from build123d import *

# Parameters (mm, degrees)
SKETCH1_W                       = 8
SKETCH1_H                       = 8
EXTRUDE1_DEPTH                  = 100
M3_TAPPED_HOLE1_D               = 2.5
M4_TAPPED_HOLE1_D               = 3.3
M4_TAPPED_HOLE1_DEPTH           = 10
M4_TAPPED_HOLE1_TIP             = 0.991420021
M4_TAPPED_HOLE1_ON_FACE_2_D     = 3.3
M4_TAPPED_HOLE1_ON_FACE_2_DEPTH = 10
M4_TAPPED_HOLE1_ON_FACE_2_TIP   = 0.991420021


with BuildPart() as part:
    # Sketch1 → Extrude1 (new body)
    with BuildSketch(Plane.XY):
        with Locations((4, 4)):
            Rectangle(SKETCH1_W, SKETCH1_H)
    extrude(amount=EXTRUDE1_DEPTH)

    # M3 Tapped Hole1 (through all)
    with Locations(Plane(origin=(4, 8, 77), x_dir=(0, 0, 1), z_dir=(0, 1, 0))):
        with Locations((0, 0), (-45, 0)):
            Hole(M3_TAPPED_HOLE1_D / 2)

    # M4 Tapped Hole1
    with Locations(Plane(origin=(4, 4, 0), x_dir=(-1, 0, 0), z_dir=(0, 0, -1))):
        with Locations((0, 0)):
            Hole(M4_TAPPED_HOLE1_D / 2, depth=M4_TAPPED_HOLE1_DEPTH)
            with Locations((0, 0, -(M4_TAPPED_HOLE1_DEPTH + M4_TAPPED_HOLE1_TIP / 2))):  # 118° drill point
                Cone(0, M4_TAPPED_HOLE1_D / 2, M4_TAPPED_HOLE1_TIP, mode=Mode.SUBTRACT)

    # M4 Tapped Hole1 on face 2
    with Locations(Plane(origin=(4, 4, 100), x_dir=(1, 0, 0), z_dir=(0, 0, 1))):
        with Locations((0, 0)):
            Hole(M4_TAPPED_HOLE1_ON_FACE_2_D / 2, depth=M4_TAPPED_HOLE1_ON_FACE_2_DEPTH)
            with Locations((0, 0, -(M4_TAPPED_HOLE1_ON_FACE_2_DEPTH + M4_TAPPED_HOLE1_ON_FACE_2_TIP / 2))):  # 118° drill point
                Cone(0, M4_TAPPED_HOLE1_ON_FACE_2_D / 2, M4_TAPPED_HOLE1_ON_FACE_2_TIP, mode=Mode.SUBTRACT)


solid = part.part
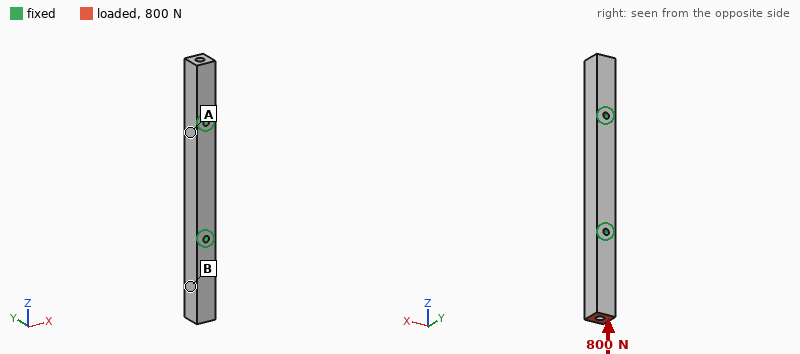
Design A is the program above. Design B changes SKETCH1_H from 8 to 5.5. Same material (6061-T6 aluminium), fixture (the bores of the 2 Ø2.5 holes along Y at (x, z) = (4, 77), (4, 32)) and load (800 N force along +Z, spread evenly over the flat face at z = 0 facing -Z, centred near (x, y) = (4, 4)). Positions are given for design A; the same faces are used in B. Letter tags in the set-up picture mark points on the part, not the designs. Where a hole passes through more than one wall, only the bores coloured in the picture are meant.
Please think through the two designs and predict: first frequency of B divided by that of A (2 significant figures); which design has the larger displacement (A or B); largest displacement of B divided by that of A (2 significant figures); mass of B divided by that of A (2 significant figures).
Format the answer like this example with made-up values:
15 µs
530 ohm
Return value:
0.86
B
1.5
0.68
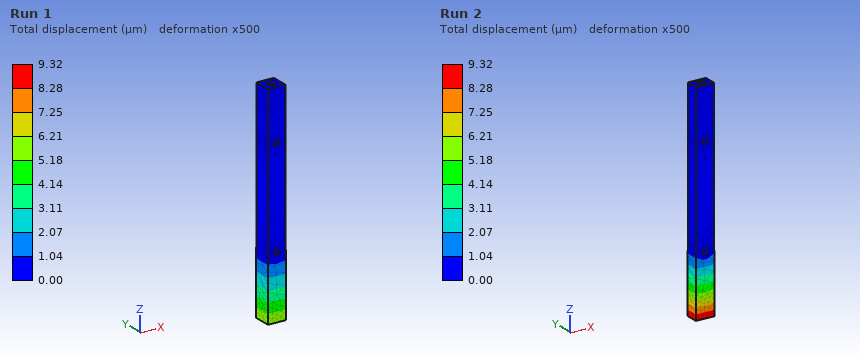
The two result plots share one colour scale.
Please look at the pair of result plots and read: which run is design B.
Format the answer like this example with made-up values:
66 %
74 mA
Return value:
Run 2
